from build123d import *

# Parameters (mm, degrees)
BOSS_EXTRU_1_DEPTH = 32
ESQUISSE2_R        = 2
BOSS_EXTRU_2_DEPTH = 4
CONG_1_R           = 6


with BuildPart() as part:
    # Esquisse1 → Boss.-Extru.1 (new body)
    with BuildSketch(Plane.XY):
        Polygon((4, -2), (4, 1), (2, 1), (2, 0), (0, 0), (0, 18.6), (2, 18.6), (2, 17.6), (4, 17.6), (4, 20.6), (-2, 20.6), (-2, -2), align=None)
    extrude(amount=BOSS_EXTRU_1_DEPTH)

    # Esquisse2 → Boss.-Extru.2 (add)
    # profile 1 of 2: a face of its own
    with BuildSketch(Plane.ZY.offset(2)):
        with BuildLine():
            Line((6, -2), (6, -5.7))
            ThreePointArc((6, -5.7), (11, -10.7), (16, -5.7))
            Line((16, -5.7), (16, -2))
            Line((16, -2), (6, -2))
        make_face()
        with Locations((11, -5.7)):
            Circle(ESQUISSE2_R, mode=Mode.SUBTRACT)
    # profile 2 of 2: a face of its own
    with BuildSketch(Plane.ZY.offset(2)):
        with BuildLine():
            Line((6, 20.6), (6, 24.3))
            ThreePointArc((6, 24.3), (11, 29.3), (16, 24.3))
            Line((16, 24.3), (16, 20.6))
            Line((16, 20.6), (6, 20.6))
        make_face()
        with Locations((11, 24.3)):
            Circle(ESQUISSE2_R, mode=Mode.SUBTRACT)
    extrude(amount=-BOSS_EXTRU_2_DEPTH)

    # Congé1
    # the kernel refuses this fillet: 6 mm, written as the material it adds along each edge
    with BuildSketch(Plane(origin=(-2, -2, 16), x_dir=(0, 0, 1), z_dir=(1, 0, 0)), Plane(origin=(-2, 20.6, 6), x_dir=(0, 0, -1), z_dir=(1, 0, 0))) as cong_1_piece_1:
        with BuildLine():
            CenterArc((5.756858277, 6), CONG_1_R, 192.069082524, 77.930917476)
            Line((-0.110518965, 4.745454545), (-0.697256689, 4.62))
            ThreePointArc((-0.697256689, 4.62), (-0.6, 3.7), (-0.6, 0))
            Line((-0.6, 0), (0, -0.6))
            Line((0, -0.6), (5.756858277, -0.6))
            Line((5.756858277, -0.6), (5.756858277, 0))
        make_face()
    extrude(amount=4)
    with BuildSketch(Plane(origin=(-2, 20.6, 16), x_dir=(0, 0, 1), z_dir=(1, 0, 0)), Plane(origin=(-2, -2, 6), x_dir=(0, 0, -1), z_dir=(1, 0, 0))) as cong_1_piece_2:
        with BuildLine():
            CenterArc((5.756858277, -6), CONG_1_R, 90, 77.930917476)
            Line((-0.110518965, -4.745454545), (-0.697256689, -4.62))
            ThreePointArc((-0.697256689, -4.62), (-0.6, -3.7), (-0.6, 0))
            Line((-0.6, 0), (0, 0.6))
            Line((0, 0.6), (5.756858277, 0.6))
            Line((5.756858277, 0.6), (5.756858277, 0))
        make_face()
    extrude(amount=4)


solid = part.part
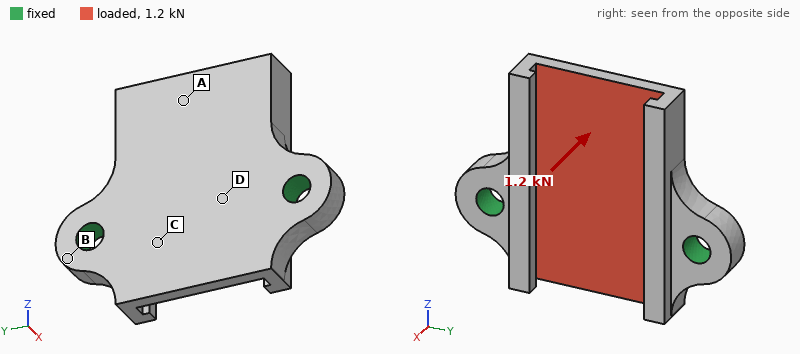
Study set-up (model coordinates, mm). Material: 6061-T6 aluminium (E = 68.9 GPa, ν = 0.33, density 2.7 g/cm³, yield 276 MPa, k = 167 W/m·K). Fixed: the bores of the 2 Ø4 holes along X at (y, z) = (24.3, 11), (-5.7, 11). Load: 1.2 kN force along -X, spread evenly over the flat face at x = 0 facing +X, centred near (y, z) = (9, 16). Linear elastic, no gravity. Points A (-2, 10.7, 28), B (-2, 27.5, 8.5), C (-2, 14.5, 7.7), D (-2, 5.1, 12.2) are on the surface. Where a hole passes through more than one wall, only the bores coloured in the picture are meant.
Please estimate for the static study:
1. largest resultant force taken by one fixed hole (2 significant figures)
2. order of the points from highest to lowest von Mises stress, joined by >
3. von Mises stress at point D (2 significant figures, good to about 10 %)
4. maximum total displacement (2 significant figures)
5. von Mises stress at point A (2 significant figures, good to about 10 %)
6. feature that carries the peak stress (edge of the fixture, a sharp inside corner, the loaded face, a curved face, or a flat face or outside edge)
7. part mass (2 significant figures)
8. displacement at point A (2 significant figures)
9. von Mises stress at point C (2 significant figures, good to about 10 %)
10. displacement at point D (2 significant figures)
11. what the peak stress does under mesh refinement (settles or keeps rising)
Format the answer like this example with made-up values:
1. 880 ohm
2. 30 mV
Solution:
1. 690 N
2. A > D > C > B
3. 64 MPa
4. 0.17 mm
5. 94 MPa
6. edge of the fixture
7. 7.3 g
8. 0.14 mm
9. 43 MPa
10. 0.035 mm
11. keeps rising
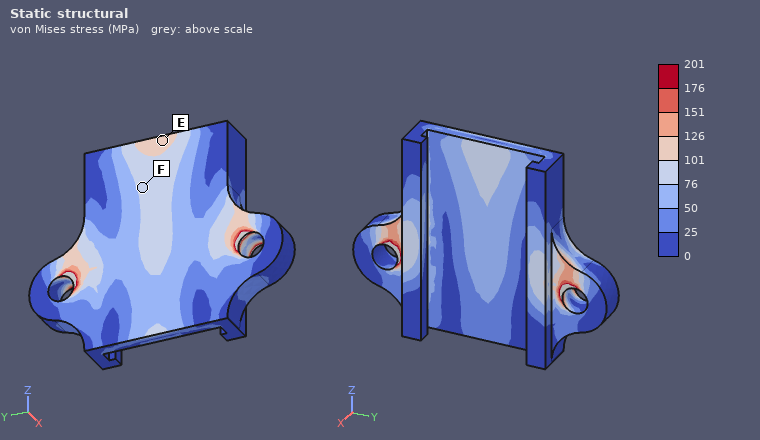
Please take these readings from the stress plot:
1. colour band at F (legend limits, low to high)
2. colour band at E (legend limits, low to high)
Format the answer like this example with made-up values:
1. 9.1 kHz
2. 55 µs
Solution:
1. 76 to 101 MPa
2. 101 to 126 MPa
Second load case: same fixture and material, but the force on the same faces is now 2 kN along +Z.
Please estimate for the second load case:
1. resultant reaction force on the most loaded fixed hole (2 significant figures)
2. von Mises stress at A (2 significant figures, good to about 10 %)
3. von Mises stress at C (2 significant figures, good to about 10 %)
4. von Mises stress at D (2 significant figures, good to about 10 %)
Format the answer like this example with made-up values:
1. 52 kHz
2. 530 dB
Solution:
1. 1.0 kN
2. 20 MPa
3. 17 MPa
4. 12 MPa
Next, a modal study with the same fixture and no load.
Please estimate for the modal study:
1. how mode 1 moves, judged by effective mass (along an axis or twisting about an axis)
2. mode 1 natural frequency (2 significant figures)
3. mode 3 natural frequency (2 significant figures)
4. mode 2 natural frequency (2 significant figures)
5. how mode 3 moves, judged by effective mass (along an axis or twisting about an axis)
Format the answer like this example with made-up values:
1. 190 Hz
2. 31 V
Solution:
1. along X
2. 7700 Hz
3. 17 kHz
4. 13 kHz
5. along X
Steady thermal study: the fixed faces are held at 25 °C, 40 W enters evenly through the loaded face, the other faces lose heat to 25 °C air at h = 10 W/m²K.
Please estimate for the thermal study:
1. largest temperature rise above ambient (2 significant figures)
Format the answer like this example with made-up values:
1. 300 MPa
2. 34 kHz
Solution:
1. 35 K
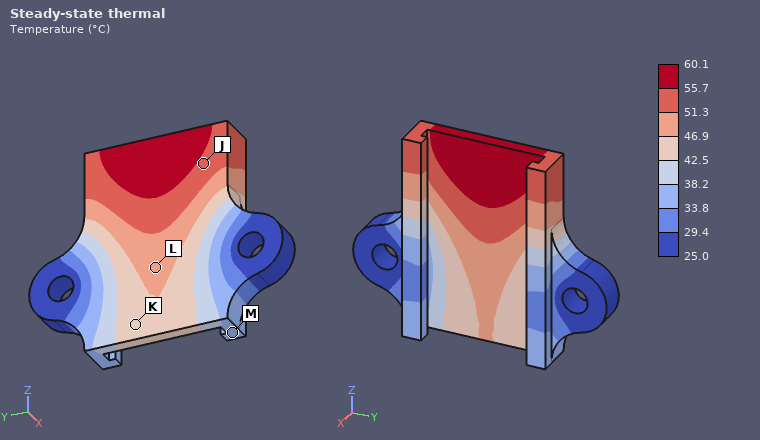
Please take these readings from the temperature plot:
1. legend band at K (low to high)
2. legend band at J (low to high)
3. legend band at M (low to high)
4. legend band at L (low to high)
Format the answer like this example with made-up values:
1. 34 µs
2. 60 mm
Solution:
1. 42.5 to 46.9 °C
2. 51.3 to 55.7 °C
3. 33.8 to 38.2 °C
4. 46.9 to 51.3 °C
